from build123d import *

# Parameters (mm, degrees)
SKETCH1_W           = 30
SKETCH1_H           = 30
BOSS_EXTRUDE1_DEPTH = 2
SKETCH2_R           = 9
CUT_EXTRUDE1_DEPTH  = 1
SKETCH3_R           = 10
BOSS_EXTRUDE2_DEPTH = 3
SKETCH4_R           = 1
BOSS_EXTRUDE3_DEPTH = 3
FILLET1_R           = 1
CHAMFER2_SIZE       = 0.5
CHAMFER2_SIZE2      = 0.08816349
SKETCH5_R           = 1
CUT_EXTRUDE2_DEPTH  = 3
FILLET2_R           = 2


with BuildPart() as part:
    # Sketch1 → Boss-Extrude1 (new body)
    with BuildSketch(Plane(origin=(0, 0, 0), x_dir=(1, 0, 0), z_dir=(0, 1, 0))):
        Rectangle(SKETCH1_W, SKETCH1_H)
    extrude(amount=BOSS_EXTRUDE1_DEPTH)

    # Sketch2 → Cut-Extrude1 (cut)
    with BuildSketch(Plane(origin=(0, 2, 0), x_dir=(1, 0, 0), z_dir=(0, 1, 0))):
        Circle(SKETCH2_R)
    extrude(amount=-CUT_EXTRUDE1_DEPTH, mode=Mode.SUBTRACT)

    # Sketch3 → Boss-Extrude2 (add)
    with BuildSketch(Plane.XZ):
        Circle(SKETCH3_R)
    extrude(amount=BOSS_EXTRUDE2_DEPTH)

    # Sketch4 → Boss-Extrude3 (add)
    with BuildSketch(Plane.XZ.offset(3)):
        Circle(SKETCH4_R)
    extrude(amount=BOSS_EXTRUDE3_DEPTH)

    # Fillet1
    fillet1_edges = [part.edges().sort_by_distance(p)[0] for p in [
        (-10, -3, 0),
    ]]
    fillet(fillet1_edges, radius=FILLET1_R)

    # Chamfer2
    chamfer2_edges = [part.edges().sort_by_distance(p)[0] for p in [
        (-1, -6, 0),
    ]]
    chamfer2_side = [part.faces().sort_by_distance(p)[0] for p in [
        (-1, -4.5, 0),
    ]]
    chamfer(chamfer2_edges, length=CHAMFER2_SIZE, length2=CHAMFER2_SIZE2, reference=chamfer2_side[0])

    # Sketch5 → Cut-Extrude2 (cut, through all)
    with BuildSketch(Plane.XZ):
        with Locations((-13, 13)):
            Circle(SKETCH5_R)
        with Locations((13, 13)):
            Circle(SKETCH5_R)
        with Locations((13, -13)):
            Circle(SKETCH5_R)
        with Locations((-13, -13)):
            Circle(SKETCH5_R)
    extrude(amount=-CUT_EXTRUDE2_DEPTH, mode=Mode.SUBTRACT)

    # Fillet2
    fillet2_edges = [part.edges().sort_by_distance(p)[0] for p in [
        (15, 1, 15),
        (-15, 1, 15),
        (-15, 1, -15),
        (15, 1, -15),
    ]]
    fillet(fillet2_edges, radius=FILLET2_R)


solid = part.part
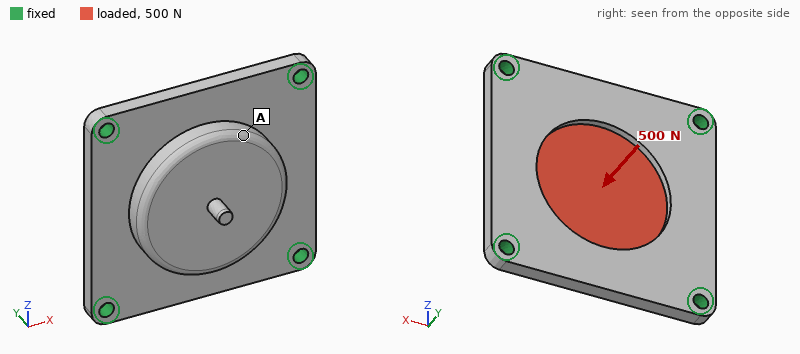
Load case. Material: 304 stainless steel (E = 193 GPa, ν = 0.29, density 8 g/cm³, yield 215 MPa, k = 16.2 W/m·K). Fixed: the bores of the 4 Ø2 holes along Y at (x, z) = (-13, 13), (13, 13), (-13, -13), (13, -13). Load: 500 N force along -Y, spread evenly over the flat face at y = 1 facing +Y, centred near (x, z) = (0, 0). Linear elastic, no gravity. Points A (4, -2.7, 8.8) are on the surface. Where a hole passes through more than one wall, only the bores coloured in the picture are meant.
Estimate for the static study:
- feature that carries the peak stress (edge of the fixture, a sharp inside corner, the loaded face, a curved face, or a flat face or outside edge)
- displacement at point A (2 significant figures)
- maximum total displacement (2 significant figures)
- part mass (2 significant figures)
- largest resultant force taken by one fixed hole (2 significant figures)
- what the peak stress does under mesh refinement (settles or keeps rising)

edge of the fixture
9.0 µm
10 µm
20 g
170 N
keeps rising
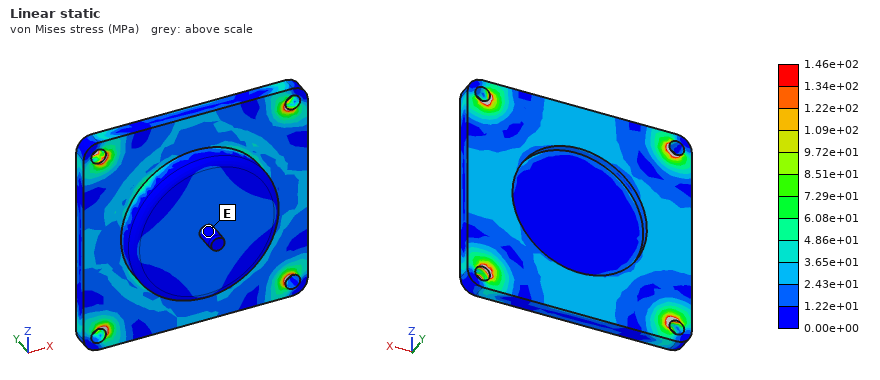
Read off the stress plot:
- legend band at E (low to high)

0.00e+00 to 1.22e+01 MPa
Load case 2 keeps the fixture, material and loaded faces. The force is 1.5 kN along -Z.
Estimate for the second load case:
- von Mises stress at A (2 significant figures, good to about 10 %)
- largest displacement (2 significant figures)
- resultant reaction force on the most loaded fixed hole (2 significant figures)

9.9 MPa
2.9 µm
410 N
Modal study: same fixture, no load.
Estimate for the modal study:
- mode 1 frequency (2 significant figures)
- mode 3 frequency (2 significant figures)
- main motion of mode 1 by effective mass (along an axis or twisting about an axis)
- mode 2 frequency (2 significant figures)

9800 Hz
16 kHz
along Y
16 kHz
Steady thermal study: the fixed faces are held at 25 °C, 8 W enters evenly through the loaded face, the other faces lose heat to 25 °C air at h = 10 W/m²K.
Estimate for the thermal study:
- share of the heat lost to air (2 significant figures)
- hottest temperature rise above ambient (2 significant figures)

9.9 %
68 K
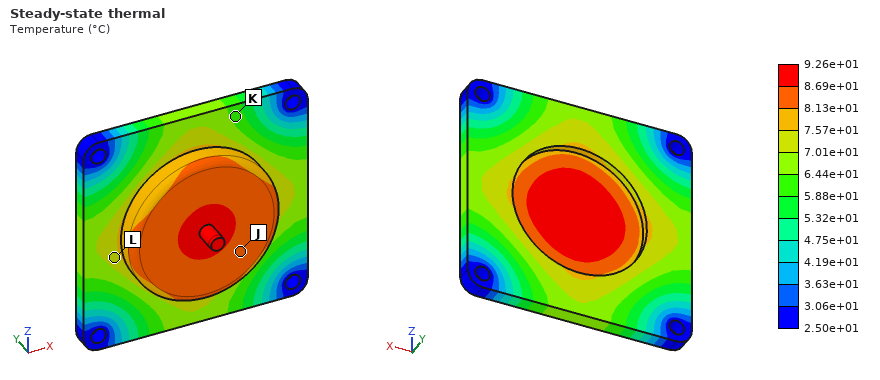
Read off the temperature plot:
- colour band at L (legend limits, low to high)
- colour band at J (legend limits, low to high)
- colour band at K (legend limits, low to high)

7.01e+01 to 7.57e+01 °C
8.13e+01 to 8.69e+01 °C
5.88e+01 to 6.44e+01 °C
